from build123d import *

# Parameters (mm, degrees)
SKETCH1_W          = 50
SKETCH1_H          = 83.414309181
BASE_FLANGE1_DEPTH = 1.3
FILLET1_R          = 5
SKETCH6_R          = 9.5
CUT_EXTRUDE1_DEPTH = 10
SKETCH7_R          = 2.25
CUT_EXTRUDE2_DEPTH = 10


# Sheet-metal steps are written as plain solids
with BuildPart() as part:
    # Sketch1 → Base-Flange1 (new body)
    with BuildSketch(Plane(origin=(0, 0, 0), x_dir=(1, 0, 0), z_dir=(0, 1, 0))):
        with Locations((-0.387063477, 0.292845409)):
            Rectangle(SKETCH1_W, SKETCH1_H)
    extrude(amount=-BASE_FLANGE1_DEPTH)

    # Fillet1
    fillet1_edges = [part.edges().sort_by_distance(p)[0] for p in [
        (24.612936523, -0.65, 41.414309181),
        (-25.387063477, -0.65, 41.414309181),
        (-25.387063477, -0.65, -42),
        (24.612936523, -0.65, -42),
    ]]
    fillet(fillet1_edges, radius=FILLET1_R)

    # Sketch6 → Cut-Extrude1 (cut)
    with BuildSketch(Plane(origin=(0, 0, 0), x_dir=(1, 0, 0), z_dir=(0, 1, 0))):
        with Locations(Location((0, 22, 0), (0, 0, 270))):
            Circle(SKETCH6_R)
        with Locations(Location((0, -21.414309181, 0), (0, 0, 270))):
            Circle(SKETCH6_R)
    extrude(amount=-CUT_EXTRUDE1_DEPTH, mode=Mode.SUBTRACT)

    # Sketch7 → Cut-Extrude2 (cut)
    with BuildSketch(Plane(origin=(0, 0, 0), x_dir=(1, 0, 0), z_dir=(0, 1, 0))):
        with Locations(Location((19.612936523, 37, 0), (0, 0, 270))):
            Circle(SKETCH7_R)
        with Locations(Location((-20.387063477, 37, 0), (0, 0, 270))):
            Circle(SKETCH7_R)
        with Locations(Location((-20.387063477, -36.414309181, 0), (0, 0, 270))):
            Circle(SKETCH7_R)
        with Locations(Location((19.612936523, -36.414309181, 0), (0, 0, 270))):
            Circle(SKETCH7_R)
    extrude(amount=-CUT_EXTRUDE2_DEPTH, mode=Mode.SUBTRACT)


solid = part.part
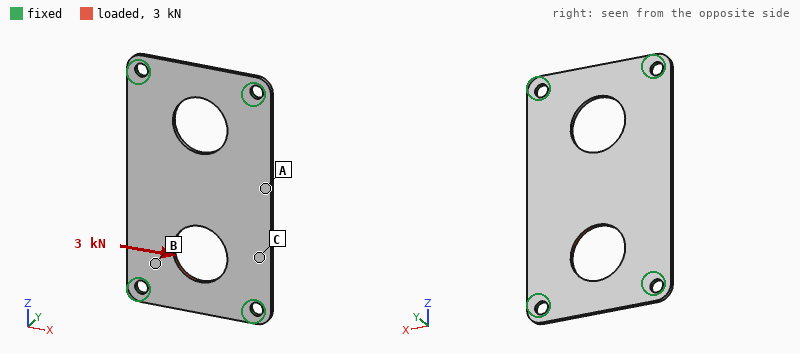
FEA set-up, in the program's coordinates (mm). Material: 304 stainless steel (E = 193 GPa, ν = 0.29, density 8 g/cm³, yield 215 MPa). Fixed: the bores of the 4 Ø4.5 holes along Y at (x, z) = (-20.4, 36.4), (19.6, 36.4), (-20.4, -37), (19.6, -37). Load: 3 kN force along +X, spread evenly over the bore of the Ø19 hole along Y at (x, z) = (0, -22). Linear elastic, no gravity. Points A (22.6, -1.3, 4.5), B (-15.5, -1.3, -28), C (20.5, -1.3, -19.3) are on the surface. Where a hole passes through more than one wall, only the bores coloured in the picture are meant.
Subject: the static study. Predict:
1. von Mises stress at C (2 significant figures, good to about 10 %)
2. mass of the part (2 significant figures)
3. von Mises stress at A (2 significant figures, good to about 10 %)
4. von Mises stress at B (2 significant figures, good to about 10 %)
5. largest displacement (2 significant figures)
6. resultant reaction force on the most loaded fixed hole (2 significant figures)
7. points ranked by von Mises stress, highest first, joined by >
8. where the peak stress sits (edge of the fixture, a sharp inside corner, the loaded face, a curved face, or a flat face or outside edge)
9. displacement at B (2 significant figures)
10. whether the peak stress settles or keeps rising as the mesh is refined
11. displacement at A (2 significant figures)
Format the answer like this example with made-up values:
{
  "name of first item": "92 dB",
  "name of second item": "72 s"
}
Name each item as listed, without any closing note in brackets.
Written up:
{
  "von Mises stress at C": "36 MPa",
  "mass of the part": "37 g",
  "von Mises stress at A": "15 MPa",
  "von Mises stress at B": "70 MPa",
  "largest displacement": "18 µm",
  "resultant reaction force on the most loaded fixed hole": "1.3 kN",
  "points ranked by von Mises stress, highest first, joined by >": "B > C > A",
  "where the peak stress sits": "edge of the fixture",
  "displacement at B": "7.4 µm",
  "whether the peak stress settles or keeps rising as the mesh is refined": "keeps rising",
  "displacement at A": "13 µm"
}
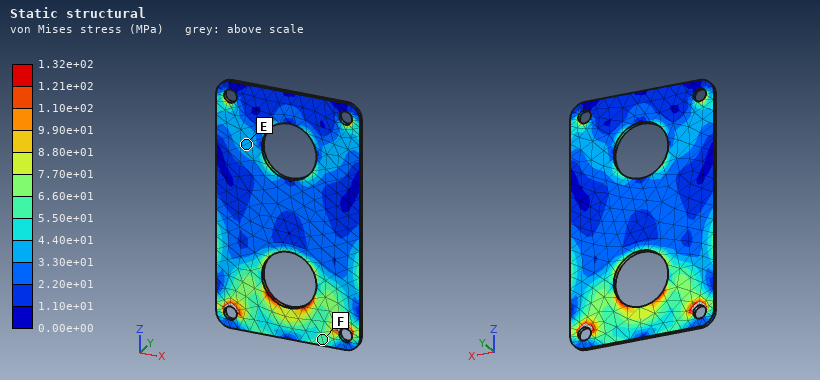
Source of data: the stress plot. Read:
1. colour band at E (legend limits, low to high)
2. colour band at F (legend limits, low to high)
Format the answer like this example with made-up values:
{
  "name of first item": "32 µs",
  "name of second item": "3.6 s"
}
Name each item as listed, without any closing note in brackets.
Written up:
{
  "colour band at E": "3.30e+01 to 4.40e+01 MPa",
  "colour band at F": "5.50e+01 to 6.60e+01 MPa"
}
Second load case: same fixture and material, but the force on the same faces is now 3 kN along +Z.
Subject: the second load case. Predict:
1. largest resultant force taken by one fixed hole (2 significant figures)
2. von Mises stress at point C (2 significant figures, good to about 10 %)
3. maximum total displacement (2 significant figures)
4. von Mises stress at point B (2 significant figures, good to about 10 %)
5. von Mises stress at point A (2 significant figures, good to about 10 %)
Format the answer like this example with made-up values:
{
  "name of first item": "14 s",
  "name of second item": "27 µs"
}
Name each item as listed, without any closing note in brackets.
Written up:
{
  "largest resultant force taken by one fixed hole": "1.1 kN",
  "von Mises stress at point C": "30 MPa",
  "maximum total displacement": "12 µm",
  "von Mises stress at point B": "50 MPa",
  "von Mises stress at point A": "16 MPa"
}
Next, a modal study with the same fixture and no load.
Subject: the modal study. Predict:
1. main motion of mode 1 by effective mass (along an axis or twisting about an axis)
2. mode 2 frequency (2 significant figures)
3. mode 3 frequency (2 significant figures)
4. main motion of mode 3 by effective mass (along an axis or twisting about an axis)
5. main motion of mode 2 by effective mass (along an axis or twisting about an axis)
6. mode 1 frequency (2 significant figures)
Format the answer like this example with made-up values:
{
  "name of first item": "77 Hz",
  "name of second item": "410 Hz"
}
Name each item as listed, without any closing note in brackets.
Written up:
{
  "main motion of mode 1 by effective mass": "along Y",
  "mode 2 frequency": "1700 Hz",
  "mode 3 frequency": "3300 Hz",
  "main motion of mode 3 by effective mass": "twisting about X",
  "main motion of mode 2 by effective mass": "twisting about Z",
  "mode 1 frequency": "1200 Hz"
}
